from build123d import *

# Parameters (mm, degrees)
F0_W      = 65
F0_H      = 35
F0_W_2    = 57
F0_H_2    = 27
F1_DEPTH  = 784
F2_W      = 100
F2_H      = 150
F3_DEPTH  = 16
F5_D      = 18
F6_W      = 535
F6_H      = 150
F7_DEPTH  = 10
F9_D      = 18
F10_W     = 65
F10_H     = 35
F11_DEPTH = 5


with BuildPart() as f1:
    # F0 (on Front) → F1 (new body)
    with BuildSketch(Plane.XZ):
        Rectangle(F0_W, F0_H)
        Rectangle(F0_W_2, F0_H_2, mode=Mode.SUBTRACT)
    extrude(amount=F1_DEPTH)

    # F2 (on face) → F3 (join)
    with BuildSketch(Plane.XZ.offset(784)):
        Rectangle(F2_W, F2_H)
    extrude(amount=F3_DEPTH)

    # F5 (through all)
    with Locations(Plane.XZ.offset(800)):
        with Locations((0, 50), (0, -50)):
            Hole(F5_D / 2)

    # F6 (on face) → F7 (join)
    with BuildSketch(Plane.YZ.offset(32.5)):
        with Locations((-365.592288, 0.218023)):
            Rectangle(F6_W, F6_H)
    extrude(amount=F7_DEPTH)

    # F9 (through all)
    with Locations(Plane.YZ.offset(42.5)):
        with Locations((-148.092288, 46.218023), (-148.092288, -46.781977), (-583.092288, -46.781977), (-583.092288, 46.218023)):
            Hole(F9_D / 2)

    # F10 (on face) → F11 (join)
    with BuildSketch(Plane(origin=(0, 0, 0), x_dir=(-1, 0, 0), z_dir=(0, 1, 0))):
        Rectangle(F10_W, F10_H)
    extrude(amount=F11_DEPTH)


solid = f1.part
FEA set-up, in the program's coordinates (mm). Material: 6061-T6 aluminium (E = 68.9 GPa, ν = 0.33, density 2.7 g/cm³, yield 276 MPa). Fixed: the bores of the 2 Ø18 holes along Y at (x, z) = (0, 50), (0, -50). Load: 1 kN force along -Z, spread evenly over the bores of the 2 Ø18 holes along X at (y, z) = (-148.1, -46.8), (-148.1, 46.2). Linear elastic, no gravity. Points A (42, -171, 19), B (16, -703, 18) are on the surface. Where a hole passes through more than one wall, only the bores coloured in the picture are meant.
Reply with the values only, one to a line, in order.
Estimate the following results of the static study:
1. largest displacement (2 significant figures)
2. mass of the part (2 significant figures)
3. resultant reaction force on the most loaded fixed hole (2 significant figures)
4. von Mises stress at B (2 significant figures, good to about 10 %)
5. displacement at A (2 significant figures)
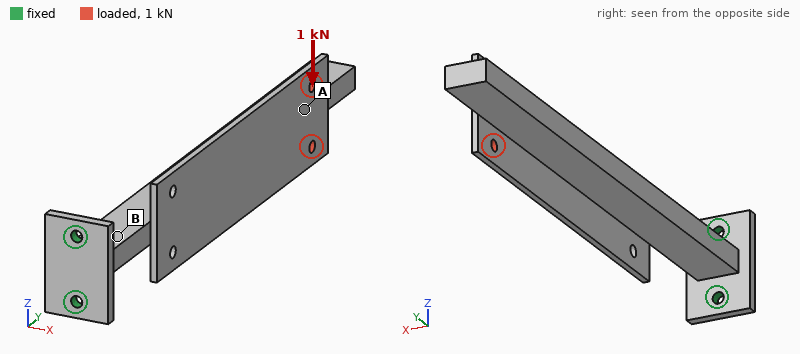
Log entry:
9.0 mm
4.4 kg
8.7 kN
73 MPa
6.7 mm
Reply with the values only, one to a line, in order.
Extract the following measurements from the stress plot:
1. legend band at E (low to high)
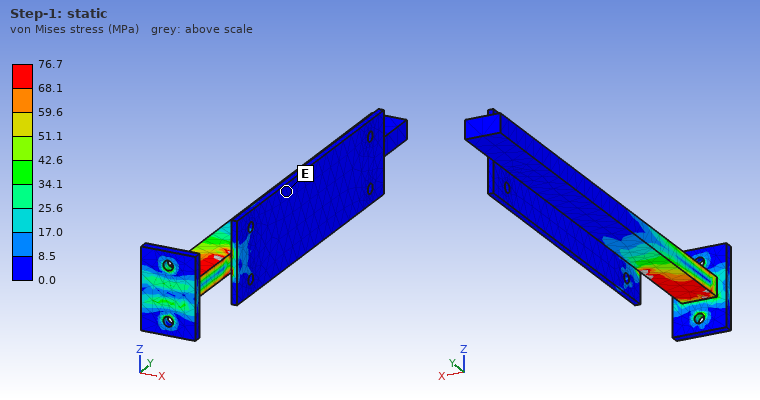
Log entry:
0.0 to 8.5 MPa
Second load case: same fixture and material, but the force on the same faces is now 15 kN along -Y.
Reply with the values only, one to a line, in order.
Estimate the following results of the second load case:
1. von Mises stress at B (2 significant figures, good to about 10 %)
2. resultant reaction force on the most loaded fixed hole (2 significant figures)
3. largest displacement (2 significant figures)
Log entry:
43 MPa
7.6 kN
4.9 mm
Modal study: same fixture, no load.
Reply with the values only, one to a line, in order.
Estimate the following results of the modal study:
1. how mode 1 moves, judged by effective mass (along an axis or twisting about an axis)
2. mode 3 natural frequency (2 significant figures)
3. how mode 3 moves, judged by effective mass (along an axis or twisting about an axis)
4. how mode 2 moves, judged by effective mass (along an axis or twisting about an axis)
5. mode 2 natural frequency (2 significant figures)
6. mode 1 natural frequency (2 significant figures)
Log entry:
along Z
340 Hz
twisting about Y
along X
58 Hz
45 Hz
